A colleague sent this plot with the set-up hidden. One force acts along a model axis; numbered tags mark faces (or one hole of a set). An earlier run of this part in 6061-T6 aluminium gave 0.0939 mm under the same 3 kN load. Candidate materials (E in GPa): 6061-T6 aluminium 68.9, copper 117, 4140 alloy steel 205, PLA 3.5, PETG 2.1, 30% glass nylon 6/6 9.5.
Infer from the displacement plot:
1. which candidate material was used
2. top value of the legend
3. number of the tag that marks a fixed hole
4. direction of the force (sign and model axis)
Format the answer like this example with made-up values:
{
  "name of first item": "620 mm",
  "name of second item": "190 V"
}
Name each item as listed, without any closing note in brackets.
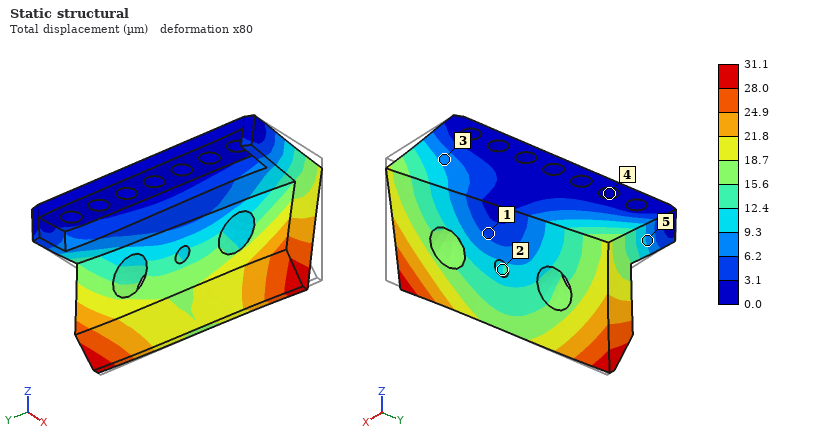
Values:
{
  "which candidate material was used": "4140 alloy steel",
  "top value of the legend": "31.1 µm",
  "number of the tag that marks a fixed hole": "4",
  "direction of the force": "+Y"
}
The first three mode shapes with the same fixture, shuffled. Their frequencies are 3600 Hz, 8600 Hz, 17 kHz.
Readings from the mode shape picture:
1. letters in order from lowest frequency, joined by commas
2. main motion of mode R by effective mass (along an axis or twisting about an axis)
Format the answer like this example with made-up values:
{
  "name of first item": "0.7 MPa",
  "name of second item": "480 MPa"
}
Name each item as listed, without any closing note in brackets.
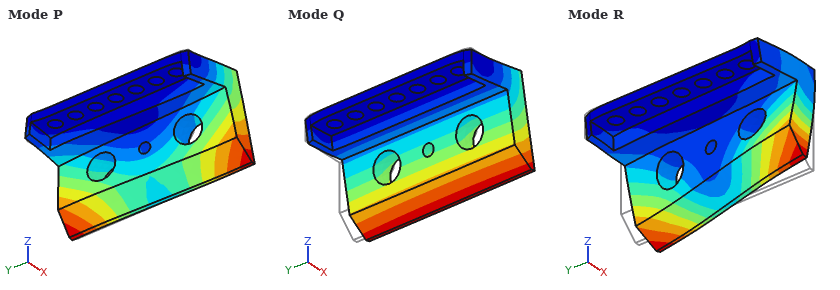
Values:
{
  "letters in order from lowest frequency, joined by commas": "Q, P, R",
  "main motion of mode R by effective mass": "along Y"
}
